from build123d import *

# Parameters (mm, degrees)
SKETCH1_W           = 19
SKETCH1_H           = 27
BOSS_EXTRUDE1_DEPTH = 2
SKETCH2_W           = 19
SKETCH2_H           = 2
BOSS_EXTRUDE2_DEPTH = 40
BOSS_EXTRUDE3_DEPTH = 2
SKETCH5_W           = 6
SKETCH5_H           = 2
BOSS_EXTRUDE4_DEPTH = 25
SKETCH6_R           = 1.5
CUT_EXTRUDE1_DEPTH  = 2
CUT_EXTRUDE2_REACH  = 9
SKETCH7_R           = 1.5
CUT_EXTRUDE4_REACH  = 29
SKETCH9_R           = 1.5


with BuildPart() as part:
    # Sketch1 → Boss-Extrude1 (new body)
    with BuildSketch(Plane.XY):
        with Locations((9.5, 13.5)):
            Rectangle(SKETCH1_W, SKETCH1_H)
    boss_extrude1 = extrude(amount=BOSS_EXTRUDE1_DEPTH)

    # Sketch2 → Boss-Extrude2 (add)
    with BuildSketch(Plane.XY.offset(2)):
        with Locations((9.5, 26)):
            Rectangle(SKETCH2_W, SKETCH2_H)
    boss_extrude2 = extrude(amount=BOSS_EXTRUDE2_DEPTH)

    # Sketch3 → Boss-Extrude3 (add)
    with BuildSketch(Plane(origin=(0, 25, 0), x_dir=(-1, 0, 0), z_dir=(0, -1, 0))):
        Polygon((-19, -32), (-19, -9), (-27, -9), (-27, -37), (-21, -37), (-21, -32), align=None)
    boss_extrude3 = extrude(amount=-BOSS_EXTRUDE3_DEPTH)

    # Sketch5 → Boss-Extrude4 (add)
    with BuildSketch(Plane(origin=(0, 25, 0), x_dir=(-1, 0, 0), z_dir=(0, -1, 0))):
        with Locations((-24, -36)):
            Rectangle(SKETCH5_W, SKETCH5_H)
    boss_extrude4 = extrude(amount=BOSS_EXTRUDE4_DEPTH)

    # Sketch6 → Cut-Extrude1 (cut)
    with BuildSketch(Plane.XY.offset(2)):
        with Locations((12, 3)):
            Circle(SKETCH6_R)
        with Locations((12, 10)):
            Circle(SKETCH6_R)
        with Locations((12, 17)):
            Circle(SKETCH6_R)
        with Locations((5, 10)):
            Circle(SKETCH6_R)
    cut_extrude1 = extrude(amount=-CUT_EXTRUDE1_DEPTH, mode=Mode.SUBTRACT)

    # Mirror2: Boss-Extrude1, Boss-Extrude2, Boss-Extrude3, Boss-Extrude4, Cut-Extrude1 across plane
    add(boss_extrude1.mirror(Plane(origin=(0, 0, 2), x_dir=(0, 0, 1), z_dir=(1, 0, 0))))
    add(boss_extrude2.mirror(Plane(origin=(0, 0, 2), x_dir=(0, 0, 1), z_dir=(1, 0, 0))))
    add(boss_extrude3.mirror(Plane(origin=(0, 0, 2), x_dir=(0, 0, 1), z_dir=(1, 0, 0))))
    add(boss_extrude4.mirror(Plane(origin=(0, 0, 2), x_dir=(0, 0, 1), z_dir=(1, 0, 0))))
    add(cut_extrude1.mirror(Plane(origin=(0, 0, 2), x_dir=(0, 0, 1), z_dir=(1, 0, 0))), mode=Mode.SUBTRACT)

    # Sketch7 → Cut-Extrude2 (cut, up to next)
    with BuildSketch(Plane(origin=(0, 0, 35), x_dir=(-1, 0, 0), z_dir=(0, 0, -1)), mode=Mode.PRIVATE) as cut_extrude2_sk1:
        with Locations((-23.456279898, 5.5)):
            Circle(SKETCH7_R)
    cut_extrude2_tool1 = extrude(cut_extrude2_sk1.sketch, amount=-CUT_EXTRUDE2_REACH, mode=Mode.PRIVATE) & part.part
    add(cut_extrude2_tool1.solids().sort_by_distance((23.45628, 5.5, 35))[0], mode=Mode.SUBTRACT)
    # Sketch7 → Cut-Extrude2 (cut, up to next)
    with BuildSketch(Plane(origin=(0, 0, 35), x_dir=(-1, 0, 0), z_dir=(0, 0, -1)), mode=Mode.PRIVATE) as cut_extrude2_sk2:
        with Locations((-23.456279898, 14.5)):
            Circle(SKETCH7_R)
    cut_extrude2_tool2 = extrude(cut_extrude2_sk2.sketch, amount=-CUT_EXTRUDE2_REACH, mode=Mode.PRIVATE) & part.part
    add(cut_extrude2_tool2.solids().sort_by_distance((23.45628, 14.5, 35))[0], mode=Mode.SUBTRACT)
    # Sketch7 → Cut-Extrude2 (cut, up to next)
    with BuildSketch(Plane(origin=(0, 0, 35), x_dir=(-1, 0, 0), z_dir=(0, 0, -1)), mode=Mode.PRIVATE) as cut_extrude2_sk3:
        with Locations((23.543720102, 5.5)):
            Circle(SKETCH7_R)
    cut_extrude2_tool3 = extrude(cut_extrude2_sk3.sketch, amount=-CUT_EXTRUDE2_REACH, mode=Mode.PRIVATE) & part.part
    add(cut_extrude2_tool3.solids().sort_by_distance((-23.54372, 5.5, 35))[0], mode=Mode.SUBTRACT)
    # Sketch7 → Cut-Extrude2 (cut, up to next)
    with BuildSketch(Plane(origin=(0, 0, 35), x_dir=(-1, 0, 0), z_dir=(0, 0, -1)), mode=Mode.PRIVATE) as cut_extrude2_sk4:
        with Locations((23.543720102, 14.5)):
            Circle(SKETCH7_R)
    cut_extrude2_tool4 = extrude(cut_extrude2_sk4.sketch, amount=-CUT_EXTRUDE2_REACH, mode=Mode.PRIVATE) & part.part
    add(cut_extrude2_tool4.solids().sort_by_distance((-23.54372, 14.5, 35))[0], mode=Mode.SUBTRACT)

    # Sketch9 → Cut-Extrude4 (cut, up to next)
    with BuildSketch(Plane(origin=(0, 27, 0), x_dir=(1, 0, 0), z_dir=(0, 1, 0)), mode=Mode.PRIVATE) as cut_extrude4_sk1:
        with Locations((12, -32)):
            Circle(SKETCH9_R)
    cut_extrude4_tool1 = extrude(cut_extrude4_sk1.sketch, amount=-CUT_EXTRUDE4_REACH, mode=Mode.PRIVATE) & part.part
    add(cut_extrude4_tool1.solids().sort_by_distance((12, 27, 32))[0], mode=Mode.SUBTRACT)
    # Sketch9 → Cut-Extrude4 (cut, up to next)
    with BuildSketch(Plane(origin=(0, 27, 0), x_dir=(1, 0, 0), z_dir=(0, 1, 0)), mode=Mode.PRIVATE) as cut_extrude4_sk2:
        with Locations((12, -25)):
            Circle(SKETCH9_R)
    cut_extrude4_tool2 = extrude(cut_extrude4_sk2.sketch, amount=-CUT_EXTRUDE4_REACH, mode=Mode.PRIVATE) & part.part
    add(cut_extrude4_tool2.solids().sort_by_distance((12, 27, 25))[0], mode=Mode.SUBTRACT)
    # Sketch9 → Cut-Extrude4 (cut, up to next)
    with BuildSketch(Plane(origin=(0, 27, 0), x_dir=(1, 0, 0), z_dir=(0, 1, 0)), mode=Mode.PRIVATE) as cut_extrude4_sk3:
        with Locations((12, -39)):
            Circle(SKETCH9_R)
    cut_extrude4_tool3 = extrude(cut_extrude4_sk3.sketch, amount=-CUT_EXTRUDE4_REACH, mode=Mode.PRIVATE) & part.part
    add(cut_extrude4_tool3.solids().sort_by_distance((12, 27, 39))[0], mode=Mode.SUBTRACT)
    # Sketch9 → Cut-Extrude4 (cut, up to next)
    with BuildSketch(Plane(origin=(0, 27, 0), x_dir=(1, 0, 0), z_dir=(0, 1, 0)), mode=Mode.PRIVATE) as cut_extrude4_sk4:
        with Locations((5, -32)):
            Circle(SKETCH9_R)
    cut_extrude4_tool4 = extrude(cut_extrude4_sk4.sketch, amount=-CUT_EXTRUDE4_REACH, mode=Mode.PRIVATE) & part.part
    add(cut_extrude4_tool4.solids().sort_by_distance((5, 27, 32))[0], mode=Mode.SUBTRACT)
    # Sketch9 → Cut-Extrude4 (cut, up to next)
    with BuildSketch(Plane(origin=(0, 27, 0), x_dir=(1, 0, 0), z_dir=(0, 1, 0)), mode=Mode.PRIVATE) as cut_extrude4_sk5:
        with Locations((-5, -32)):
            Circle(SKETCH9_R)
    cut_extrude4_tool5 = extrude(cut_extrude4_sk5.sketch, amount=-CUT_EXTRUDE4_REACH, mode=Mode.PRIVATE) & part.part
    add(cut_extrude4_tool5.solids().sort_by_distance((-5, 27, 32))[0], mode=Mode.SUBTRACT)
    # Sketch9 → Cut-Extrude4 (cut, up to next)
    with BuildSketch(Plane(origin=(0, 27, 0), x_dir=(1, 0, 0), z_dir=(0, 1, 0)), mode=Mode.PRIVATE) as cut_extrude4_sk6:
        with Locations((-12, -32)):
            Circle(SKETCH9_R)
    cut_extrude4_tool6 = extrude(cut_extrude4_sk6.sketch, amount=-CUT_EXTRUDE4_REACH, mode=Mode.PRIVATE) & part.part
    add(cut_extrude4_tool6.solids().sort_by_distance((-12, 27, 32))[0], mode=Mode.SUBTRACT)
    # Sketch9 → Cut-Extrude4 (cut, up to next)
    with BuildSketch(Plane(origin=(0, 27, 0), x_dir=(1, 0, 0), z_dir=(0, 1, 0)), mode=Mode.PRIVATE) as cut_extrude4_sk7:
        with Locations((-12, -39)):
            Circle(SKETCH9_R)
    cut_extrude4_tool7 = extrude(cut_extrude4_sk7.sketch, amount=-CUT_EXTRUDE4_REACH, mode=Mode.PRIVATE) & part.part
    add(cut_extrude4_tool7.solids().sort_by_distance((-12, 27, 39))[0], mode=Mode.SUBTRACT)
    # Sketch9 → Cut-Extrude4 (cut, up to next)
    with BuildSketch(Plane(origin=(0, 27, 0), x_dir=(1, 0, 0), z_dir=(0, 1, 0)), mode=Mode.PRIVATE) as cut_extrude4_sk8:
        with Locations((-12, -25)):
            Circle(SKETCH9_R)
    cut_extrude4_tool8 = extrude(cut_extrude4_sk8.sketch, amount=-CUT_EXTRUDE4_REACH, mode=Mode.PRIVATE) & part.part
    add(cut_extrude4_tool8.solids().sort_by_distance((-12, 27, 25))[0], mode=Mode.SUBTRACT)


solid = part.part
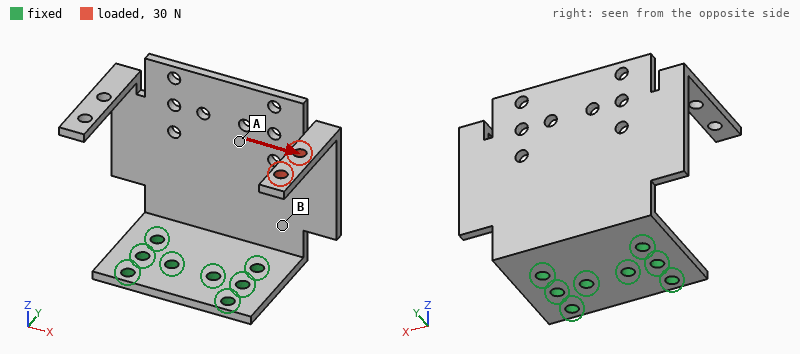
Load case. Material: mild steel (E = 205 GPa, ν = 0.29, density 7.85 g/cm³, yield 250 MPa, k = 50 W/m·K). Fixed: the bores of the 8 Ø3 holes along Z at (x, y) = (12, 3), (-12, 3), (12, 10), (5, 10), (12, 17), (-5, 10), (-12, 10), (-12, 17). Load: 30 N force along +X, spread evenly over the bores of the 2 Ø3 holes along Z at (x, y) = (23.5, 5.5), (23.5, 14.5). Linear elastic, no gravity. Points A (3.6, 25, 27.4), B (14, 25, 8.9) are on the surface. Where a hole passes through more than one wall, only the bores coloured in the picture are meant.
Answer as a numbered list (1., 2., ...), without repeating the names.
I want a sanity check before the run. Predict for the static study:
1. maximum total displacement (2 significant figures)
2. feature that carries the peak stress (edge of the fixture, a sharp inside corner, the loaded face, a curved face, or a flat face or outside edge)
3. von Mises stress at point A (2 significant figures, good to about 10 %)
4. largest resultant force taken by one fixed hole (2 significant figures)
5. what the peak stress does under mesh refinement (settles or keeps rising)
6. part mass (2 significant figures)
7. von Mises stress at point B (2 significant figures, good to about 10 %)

1. 0.20 mm
2. a sharp inside corner
3. 13 MPa
4. 52 N
5. keeps rising
6. 49 g
7. 27 MPa
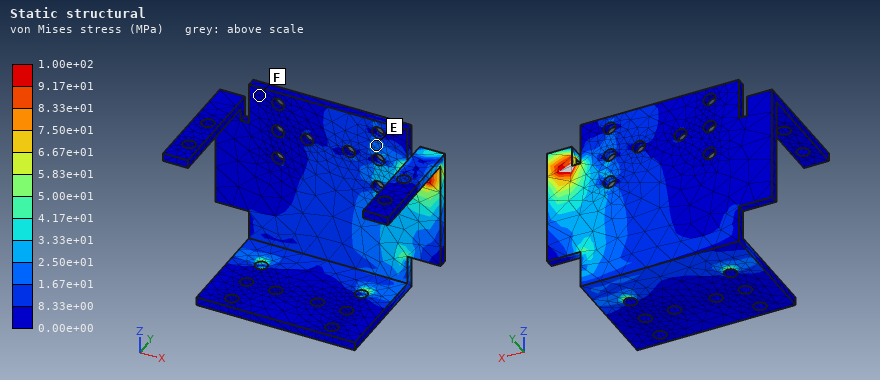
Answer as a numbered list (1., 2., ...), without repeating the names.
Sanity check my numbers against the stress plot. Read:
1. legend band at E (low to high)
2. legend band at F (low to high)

1. 1.67e+01 to 2.50e+01 MPa
2. 0.00e+00 to 8.33e+00 MPa
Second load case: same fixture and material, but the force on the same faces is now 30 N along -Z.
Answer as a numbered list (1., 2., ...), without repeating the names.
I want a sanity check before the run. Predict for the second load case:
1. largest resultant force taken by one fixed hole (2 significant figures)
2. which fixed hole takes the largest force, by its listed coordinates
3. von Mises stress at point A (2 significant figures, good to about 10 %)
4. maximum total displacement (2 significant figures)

1. 36 N
2. (12, 17)
3. 14 MPa
4. 0.33 mm
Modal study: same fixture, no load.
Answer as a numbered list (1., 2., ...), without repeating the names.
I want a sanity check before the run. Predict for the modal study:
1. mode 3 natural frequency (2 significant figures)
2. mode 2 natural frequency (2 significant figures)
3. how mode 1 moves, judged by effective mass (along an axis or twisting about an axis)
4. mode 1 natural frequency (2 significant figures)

1. 1500 Hz
2. 1000 Hz
3. along Y
4. 590 Hz
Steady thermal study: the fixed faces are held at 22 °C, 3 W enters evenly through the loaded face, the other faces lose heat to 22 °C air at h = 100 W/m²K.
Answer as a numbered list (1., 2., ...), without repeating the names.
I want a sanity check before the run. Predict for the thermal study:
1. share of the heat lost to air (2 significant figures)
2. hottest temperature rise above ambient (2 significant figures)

1. 93 %
2. 62 K
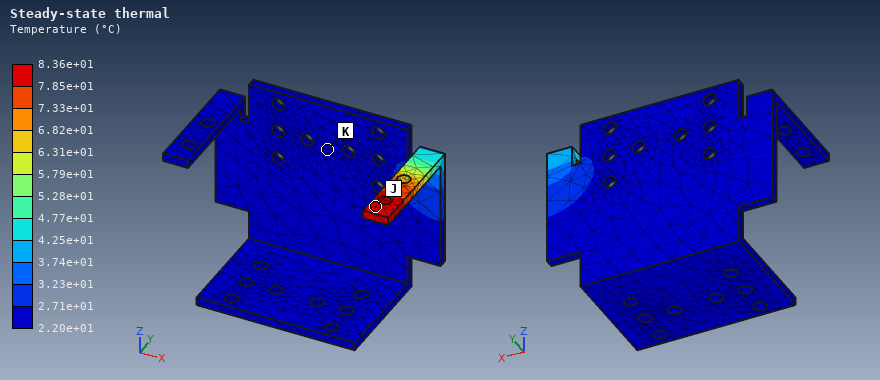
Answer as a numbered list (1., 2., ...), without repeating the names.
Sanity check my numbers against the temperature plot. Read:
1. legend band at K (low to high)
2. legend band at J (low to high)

1. 2.20e+01 to 2.71e+01 °C
2. 7.85e+01 to 8.36e+01 °C
